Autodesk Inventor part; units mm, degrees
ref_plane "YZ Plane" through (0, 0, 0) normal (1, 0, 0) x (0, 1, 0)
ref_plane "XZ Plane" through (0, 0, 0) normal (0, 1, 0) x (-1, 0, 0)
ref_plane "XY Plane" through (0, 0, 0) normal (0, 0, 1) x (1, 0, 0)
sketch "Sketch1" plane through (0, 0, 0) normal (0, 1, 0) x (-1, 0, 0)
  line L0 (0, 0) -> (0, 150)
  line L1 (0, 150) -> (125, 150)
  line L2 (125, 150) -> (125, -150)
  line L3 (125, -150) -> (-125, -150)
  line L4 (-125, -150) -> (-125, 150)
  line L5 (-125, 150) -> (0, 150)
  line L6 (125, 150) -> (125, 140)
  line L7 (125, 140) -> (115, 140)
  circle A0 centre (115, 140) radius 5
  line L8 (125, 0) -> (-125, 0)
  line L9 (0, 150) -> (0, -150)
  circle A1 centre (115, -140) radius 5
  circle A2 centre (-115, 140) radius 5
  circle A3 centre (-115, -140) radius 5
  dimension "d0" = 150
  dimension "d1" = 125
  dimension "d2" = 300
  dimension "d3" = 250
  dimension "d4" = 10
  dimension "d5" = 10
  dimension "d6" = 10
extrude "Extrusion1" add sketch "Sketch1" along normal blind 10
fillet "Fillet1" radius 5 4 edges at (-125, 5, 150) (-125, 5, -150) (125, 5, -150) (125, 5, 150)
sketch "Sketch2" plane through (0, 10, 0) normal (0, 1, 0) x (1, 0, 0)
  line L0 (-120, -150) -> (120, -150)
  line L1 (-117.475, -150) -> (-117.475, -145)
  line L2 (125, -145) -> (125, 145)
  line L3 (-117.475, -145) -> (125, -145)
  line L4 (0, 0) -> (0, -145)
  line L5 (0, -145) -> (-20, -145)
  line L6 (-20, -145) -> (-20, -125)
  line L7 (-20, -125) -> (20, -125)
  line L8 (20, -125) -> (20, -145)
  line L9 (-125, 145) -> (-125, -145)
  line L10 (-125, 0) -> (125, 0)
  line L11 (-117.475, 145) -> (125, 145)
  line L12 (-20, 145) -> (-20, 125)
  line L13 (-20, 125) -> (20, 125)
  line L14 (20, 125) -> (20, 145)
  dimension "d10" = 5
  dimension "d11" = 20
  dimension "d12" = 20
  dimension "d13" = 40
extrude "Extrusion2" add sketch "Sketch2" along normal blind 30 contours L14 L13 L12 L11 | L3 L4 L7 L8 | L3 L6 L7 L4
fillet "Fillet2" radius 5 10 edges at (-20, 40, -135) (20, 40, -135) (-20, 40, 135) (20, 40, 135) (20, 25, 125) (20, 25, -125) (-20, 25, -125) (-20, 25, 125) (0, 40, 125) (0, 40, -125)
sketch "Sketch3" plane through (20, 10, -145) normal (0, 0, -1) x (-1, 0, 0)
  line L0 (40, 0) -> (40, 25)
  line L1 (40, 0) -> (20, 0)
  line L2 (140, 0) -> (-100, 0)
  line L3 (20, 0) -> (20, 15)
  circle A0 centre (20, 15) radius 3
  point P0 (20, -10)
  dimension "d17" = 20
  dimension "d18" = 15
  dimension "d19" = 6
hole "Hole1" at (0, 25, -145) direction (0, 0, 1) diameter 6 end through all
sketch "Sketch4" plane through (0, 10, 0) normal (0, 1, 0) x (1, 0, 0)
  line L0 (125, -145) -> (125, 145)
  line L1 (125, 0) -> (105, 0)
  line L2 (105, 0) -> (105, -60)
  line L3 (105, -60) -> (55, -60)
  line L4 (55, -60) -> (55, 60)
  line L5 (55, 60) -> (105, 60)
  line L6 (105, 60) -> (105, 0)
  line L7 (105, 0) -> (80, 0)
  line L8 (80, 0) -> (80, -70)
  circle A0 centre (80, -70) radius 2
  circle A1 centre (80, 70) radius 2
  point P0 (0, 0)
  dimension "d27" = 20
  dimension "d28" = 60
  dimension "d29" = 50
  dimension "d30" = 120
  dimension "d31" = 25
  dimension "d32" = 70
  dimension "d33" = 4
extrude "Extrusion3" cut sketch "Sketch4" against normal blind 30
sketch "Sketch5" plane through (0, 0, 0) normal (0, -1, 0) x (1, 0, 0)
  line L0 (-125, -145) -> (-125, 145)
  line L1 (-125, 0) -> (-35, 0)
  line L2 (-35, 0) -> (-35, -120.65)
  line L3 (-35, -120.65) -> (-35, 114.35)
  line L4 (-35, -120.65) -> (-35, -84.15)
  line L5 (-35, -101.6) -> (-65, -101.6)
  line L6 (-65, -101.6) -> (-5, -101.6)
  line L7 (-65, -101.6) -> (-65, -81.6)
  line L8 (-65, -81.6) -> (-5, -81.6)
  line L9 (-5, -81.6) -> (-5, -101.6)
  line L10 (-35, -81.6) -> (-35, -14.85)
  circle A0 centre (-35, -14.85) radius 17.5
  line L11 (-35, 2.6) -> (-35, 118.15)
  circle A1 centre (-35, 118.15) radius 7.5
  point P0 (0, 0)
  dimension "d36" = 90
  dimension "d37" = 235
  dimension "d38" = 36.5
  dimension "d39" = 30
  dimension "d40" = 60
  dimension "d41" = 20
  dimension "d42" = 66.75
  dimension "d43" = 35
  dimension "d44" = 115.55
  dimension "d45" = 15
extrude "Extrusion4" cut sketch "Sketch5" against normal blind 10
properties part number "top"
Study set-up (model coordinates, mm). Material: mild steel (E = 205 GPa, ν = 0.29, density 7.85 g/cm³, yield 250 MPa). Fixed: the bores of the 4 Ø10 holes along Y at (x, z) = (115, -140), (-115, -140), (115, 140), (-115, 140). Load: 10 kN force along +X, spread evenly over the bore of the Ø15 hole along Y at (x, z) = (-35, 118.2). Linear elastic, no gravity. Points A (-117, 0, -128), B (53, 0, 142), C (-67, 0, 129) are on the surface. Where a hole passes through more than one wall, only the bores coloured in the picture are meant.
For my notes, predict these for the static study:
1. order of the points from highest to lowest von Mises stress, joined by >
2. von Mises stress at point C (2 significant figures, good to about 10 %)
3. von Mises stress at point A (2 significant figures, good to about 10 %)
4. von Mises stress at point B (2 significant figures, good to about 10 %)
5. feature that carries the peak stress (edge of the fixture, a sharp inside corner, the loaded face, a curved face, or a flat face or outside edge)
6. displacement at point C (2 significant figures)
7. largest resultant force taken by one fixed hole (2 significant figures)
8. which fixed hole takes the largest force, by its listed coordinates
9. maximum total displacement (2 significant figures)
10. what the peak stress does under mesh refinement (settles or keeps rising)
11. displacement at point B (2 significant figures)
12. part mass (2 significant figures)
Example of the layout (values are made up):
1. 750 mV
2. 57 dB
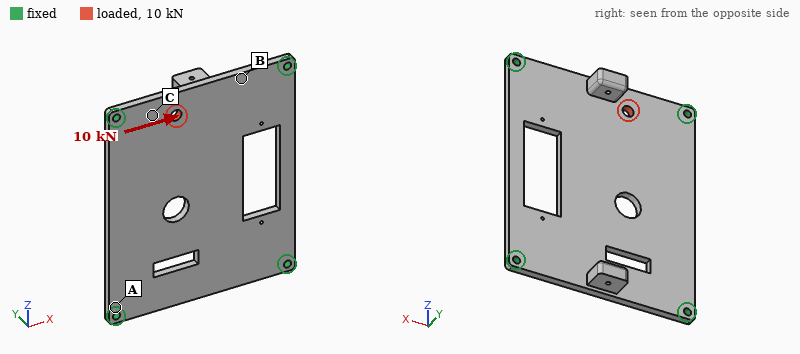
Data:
1. C > B > A
2. 14 MPa
3. 3.5 MPa
4. 8.7 MPa
5. edge of the fixture
6. 4.3 µm
7. 5.6 kN
8. (-115, 140)
9. 6.8 µm
10. keeps rising
11. 3.3 µm
12. 5.6 kg
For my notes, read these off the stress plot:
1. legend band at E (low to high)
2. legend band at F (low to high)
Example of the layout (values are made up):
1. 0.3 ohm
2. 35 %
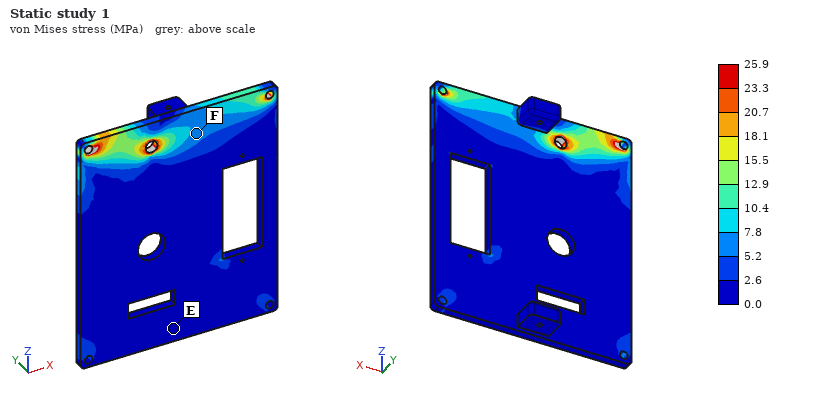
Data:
1. 0.0 to 2.6 MPa
2. 5.2 to 7.8 MPa
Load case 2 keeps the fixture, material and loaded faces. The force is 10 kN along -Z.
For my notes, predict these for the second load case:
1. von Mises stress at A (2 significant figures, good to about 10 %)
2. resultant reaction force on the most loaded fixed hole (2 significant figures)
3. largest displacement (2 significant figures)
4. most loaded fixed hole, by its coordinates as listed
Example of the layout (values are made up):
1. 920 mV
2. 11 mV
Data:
1. 11 MPa
2. 4.6 kN
3. 11 µm
4. (-115, 140)
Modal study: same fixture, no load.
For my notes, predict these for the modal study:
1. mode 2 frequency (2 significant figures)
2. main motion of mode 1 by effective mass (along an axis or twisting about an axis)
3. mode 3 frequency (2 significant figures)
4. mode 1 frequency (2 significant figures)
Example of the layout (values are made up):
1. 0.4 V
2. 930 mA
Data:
1. 820 Hz
2. along Y
3. 850 Hz
4. 450 Hz
